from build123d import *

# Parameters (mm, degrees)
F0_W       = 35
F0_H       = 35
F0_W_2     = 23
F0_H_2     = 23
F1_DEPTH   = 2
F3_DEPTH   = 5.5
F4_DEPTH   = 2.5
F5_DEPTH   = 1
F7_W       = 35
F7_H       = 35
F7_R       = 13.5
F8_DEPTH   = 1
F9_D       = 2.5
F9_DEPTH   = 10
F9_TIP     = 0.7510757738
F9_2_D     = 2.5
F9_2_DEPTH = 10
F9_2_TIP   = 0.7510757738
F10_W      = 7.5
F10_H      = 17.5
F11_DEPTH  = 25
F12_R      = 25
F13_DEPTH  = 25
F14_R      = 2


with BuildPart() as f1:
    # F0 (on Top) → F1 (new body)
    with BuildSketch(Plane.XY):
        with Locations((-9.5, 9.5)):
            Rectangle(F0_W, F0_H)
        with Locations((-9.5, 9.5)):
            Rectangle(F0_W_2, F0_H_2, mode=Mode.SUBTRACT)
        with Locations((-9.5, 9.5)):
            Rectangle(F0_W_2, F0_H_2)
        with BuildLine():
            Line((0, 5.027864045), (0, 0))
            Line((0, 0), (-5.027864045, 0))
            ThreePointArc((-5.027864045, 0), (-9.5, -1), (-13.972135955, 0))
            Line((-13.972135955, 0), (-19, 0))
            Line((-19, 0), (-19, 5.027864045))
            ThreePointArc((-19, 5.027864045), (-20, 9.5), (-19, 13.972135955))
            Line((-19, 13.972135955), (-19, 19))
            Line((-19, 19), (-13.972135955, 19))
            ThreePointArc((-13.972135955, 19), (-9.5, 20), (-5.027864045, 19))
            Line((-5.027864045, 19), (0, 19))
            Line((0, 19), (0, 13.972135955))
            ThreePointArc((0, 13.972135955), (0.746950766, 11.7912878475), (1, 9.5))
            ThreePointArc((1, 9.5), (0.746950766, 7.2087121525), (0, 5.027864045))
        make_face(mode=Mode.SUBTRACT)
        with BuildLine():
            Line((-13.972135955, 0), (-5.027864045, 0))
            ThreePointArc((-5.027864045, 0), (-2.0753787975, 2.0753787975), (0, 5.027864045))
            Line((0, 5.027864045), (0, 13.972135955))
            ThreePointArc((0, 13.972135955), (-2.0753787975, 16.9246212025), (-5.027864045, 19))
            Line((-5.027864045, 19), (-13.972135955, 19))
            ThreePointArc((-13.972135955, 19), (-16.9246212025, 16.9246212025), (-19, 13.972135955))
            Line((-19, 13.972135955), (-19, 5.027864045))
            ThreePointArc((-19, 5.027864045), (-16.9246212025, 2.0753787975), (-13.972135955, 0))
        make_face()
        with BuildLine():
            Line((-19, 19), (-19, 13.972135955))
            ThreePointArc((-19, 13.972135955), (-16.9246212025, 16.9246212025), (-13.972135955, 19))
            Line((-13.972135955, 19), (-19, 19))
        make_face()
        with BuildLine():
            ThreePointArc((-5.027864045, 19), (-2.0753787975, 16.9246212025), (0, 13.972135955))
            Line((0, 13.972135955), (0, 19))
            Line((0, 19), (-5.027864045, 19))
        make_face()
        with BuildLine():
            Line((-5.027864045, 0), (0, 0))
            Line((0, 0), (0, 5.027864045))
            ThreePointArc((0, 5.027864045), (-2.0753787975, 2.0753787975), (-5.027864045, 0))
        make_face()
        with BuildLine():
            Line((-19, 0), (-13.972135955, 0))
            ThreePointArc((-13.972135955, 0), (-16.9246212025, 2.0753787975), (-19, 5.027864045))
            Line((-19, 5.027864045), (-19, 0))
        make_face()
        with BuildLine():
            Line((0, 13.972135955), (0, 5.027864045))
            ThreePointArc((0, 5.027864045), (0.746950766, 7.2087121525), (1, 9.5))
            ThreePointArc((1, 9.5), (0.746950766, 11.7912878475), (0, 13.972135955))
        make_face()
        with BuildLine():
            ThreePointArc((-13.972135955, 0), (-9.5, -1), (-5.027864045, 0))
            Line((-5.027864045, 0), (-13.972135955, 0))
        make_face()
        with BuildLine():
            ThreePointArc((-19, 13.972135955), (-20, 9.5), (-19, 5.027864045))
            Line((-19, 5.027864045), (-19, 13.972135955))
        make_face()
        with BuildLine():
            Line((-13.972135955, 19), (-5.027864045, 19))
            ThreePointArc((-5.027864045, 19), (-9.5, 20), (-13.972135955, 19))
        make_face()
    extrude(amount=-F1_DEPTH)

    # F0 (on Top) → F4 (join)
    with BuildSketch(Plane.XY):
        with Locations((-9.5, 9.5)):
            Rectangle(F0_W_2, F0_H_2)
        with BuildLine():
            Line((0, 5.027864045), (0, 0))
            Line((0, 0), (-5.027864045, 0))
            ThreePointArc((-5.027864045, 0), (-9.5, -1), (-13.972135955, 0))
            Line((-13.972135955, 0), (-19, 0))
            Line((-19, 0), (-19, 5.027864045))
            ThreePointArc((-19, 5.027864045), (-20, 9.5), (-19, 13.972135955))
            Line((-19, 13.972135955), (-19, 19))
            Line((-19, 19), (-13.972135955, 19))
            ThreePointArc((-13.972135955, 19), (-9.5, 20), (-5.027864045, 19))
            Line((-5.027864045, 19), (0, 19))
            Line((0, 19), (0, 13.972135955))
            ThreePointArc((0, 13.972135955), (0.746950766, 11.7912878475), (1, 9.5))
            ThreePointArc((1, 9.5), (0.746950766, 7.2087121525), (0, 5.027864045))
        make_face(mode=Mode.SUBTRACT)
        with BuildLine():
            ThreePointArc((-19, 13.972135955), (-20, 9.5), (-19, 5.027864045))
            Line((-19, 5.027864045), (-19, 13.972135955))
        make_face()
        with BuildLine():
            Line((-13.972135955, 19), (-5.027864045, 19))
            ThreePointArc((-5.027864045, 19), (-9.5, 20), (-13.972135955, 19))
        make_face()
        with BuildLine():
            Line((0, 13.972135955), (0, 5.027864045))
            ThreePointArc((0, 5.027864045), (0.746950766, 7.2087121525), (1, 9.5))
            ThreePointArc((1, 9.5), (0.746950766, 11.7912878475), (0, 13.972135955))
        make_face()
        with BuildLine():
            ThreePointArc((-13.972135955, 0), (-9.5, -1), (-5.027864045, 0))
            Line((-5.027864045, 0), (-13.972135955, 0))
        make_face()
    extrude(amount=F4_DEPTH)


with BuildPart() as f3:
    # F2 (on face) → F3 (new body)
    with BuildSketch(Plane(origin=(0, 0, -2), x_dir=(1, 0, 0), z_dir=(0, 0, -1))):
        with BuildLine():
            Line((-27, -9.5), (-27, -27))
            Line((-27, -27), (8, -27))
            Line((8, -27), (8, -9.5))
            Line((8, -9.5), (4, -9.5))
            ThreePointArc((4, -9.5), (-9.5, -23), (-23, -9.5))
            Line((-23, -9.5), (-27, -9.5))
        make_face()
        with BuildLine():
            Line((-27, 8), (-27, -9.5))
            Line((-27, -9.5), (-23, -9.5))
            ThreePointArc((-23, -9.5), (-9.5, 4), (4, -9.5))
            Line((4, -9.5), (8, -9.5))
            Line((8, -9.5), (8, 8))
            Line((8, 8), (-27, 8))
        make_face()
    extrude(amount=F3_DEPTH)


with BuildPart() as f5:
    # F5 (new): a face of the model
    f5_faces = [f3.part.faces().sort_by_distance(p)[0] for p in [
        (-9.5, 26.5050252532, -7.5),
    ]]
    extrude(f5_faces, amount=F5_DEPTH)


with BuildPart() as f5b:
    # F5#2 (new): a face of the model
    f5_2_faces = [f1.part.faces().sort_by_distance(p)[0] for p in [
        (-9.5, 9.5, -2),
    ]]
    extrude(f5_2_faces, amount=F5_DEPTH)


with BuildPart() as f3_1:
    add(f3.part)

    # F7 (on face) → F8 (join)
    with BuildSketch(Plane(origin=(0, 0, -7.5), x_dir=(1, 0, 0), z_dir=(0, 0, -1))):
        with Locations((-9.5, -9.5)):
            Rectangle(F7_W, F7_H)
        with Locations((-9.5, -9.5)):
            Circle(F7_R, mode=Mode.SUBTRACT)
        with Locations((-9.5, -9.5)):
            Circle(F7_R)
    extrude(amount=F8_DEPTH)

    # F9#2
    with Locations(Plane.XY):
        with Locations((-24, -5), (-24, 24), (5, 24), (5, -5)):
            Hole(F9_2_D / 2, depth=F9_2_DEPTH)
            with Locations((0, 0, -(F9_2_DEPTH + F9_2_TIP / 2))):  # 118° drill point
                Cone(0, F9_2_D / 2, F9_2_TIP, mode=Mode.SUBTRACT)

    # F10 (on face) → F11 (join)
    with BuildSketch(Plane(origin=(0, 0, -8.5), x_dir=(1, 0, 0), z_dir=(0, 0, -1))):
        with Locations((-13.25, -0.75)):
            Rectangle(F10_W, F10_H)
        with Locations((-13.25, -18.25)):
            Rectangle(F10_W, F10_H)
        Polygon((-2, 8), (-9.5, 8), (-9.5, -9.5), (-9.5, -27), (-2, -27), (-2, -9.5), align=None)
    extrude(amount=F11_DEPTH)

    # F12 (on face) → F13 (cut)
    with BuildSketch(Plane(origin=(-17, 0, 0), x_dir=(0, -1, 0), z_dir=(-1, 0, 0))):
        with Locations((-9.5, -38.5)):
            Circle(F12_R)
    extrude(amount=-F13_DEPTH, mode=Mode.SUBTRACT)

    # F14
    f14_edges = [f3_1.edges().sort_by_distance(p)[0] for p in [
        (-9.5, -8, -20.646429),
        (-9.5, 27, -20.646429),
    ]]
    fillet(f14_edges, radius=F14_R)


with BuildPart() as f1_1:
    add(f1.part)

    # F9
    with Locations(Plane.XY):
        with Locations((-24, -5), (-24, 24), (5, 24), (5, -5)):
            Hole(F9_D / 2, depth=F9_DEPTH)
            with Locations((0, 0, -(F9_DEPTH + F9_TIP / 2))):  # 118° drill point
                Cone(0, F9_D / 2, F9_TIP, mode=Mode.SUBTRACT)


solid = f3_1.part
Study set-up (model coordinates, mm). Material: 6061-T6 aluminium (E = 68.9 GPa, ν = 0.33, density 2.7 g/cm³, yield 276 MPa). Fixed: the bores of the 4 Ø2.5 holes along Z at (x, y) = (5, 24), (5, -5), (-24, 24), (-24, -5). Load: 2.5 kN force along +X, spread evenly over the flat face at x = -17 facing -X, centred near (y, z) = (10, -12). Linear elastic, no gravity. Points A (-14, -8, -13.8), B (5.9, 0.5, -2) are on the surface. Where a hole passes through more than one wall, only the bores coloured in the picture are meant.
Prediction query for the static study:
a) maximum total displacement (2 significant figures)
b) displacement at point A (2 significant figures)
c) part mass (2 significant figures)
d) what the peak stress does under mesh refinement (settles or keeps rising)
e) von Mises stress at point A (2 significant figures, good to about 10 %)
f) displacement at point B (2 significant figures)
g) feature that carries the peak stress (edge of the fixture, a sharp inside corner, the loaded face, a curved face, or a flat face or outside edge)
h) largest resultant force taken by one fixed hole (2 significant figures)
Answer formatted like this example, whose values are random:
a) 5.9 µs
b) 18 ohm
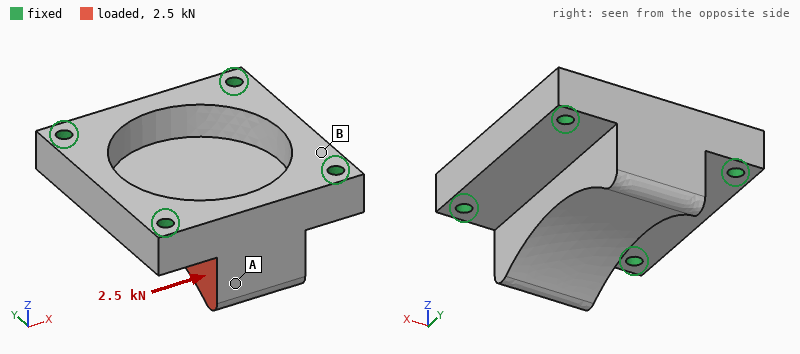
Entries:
a) 9.3 µm
b) 6.1 µm
c) 23 g
d) keeps rising
e) 11 MPa
f) 1.6 µm
g) edge of the fixture
h) 750 N
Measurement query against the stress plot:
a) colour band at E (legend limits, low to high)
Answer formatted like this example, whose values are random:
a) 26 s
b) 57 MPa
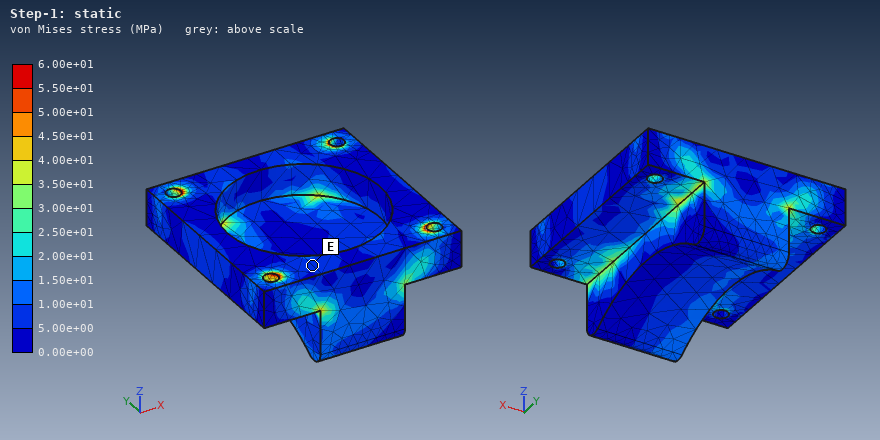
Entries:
a) 5.00e+00 to 1.00e+01 MPa
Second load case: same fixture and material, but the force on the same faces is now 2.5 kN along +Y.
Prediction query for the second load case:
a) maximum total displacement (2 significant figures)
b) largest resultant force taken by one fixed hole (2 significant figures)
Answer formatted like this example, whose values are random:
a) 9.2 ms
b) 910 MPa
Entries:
a) 18 µm
b) 820 N
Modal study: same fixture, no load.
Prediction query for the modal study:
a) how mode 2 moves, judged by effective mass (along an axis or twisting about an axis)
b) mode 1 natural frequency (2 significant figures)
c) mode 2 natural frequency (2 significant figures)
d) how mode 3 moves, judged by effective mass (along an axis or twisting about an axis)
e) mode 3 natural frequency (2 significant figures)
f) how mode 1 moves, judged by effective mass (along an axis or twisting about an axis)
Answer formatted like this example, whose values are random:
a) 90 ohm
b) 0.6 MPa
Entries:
a) along Y
b) 20 kHz
c) 23 kHz
d) along Y
e) 27 kHz
f) along Z
